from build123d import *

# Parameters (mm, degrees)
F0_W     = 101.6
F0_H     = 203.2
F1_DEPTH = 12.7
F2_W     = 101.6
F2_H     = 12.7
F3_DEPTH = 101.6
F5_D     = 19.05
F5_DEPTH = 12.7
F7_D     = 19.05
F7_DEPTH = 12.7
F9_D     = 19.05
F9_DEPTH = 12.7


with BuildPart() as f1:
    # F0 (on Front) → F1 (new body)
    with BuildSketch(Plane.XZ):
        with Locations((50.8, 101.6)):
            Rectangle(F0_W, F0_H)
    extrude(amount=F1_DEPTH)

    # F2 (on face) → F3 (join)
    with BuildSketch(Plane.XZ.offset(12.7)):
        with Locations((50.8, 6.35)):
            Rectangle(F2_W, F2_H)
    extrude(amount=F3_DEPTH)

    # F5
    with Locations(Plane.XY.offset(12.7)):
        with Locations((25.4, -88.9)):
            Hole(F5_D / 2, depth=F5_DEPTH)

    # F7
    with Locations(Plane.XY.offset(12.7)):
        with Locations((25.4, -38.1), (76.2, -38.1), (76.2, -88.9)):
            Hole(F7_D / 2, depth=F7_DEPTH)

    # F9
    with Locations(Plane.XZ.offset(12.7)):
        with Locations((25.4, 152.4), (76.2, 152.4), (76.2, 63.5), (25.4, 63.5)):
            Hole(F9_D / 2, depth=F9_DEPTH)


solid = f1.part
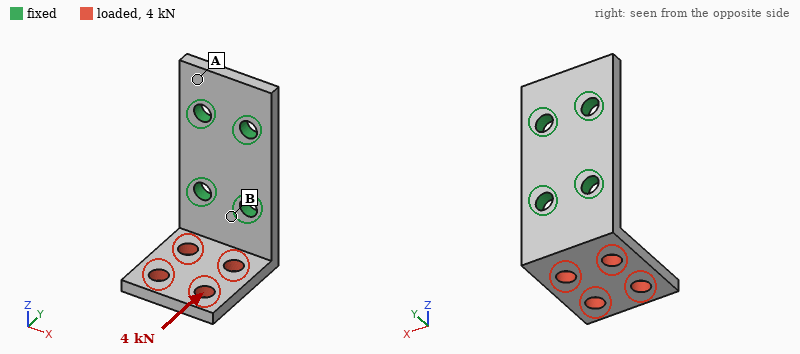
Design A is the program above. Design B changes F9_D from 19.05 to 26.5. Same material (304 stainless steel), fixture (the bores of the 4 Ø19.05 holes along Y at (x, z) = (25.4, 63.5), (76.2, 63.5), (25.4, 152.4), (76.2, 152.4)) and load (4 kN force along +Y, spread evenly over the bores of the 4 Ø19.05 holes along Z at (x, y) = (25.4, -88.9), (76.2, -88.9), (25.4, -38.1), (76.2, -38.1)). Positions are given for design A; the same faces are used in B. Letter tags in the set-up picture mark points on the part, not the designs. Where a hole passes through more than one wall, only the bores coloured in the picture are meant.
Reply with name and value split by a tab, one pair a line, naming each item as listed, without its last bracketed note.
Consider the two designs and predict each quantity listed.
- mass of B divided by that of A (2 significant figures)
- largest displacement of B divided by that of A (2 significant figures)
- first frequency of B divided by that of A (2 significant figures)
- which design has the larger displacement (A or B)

mass of B divided by that of A	0.96
largest displacement of B divided by that of A	0.83
first frequency of B divided by that of A	1.0
which design has the larger displacement	A
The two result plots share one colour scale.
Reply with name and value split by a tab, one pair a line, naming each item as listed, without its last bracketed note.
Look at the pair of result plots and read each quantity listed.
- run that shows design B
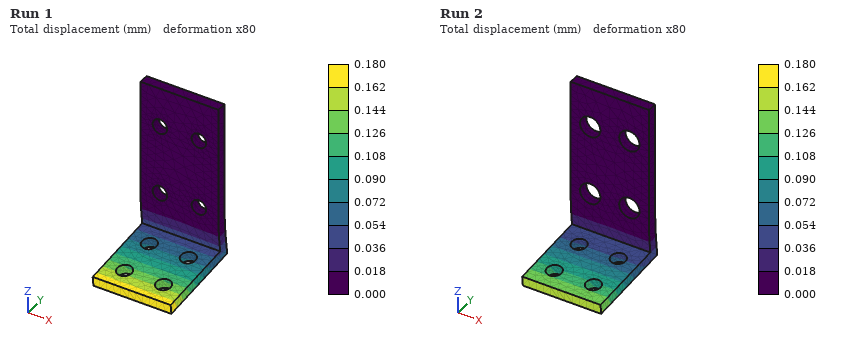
run that shows design B	Run 2
